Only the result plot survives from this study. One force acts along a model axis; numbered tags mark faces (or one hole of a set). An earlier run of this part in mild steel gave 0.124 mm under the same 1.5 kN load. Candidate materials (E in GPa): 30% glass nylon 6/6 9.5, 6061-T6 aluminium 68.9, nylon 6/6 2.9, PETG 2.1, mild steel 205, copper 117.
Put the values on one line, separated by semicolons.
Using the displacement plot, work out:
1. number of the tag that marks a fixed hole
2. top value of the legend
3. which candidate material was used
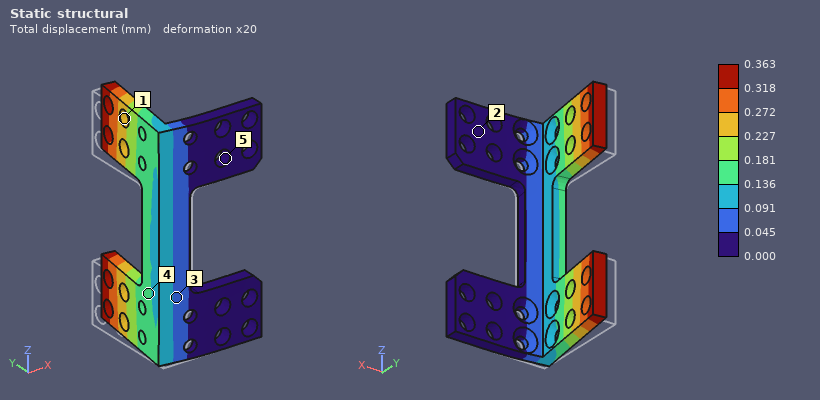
5; 0.363 mm; 6061-T6 aluminium
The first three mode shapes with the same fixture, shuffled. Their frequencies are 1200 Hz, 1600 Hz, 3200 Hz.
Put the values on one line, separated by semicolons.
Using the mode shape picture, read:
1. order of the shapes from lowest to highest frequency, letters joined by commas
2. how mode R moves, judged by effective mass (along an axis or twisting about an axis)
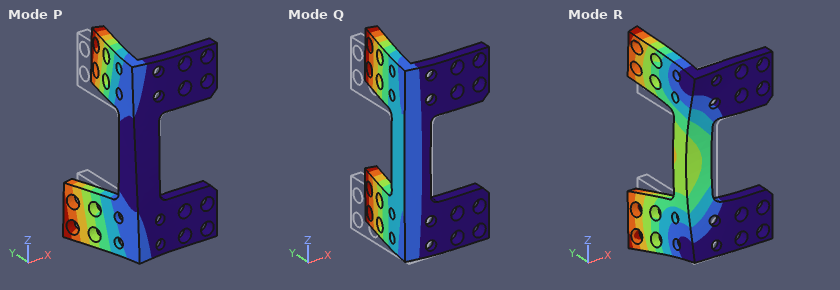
Q, P, R; along Y
